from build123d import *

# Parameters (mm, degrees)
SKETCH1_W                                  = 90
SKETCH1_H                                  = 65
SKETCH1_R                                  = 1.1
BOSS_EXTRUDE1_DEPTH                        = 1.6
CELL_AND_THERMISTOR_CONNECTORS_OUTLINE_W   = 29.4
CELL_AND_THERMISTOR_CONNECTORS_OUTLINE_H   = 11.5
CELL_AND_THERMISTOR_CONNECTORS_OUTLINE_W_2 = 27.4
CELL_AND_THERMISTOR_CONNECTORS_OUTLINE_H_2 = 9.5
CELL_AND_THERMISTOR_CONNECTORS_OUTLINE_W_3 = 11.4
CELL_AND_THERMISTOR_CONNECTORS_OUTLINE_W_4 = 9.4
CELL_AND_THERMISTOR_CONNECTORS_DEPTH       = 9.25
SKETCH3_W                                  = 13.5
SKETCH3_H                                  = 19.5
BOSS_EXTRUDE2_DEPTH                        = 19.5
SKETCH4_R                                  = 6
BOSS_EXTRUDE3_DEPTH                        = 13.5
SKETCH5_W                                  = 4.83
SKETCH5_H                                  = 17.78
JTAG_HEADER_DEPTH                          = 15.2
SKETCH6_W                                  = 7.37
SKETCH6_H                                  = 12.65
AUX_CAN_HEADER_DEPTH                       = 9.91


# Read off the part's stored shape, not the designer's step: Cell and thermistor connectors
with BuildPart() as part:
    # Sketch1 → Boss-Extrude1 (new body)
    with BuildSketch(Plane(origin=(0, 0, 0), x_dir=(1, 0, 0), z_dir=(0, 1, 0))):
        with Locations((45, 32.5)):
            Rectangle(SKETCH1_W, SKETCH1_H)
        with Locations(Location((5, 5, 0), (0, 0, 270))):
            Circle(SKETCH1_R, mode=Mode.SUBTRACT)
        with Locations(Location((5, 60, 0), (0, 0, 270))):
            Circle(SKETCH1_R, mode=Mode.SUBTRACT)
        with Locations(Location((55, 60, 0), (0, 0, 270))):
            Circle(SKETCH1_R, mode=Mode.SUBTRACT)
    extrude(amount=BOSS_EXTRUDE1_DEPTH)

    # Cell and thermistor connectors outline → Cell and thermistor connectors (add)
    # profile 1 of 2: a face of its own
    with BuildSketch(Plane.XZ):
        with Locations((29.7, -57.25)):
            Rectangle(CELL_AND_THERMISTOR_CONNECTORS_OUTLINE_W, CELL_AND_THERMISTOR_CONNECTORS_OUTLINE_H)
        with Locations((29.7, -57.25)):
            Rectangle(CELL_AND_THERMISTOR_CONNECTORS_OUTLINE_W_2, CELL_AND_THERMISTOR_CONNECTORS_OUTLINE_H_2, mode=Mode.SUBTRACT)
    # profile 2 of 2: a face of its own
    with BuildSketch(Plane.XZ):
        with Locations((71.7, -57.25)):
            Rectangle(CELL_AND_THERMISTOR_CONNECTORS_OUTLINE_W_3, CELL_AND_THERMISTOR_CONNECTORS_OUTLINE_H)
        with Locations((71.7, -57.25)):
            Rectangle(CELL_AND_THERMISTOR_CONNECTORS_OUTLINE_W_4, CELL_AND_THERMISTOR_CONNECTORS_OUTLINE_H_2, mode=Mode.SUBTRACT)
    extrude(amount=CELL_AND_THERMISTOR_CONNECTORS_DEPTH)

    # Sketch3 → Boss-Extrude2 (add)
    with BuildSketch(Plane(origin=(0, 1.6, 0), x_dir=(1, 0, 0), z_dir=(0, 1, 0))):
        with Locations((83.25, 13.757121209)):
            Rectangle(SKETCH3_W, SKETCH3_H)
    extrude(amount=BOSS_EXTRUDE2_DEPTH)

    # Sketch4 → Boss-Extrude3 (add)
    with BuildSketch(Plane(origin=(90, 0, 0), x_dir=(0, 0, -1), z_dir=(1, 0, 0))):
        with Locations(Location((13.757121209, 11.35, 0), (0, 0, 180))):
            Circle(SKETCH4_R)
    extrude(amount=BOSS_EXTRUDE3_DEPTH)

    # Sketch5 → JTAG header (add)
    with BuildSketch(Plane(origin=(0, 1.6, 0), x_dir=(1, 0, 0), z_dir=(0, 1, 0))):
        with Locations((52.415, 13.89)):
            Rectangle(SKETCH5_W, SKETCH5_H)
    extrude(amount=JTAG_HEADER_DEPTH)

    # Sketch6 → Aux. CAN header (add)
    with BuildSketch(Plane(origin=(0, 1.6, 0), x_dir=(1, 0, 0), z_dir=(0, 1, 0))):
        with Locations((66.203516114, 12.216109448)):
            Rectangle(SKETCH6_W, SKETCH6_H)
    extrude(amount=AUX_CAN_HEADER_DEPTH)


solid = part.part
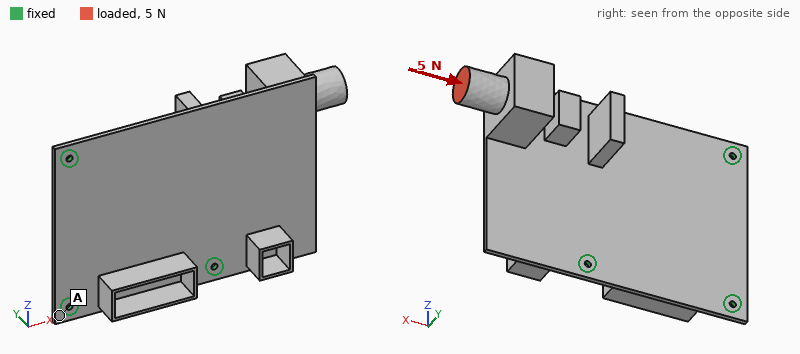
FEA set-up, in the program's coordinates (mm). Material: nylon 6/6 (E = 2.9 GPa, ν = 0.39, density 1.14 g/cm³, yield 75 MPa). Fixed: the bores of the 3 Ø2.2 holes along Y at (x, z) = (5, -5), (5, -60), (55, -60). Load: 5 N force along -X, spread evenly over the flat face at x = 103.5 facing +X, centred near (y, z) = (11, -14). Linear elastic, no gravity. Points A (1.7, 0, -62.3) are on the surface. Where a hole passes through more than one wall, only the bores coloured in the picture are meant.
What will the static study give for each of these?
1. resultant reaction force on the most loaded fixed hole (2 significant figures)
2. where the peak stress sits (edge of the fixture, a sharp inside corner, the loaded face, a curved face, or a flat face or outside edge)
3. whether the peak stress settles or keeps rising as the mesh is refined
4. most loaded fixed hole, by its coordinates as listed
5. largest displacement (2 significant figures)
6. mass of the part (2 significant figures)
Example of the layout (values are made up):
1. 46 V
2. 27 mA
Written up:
1. 3.2 N
2. edge of the fixture
3. keeps rising
4. (5, -5)
5. 1.3 mm
6. 22 g
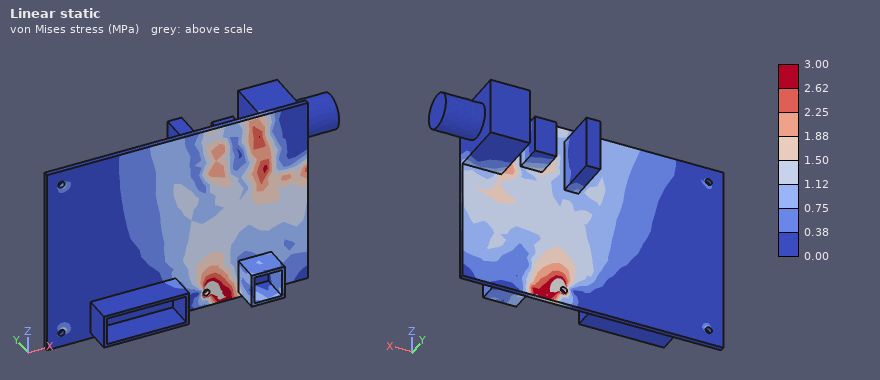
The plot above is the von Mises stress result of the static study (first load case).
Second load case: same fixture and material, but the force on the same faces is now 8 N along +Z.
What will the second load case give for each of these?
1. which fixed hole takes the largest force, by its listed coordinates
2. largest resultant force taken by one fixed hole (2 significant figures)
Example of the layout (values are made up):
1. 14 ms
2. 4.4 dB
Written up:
1. (55, -60)
2. 11 N
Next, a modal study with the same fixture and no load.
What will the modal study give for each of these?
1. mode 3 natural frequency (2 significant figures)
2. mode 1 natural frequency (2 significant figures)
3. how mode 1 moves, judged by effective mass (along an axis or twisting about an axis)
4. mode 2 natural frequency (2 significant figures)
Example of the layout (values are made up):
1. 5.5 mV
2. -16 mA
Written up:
1. 320 Hz
2. 55 Hz
3. along Y
4. 180 Hz
